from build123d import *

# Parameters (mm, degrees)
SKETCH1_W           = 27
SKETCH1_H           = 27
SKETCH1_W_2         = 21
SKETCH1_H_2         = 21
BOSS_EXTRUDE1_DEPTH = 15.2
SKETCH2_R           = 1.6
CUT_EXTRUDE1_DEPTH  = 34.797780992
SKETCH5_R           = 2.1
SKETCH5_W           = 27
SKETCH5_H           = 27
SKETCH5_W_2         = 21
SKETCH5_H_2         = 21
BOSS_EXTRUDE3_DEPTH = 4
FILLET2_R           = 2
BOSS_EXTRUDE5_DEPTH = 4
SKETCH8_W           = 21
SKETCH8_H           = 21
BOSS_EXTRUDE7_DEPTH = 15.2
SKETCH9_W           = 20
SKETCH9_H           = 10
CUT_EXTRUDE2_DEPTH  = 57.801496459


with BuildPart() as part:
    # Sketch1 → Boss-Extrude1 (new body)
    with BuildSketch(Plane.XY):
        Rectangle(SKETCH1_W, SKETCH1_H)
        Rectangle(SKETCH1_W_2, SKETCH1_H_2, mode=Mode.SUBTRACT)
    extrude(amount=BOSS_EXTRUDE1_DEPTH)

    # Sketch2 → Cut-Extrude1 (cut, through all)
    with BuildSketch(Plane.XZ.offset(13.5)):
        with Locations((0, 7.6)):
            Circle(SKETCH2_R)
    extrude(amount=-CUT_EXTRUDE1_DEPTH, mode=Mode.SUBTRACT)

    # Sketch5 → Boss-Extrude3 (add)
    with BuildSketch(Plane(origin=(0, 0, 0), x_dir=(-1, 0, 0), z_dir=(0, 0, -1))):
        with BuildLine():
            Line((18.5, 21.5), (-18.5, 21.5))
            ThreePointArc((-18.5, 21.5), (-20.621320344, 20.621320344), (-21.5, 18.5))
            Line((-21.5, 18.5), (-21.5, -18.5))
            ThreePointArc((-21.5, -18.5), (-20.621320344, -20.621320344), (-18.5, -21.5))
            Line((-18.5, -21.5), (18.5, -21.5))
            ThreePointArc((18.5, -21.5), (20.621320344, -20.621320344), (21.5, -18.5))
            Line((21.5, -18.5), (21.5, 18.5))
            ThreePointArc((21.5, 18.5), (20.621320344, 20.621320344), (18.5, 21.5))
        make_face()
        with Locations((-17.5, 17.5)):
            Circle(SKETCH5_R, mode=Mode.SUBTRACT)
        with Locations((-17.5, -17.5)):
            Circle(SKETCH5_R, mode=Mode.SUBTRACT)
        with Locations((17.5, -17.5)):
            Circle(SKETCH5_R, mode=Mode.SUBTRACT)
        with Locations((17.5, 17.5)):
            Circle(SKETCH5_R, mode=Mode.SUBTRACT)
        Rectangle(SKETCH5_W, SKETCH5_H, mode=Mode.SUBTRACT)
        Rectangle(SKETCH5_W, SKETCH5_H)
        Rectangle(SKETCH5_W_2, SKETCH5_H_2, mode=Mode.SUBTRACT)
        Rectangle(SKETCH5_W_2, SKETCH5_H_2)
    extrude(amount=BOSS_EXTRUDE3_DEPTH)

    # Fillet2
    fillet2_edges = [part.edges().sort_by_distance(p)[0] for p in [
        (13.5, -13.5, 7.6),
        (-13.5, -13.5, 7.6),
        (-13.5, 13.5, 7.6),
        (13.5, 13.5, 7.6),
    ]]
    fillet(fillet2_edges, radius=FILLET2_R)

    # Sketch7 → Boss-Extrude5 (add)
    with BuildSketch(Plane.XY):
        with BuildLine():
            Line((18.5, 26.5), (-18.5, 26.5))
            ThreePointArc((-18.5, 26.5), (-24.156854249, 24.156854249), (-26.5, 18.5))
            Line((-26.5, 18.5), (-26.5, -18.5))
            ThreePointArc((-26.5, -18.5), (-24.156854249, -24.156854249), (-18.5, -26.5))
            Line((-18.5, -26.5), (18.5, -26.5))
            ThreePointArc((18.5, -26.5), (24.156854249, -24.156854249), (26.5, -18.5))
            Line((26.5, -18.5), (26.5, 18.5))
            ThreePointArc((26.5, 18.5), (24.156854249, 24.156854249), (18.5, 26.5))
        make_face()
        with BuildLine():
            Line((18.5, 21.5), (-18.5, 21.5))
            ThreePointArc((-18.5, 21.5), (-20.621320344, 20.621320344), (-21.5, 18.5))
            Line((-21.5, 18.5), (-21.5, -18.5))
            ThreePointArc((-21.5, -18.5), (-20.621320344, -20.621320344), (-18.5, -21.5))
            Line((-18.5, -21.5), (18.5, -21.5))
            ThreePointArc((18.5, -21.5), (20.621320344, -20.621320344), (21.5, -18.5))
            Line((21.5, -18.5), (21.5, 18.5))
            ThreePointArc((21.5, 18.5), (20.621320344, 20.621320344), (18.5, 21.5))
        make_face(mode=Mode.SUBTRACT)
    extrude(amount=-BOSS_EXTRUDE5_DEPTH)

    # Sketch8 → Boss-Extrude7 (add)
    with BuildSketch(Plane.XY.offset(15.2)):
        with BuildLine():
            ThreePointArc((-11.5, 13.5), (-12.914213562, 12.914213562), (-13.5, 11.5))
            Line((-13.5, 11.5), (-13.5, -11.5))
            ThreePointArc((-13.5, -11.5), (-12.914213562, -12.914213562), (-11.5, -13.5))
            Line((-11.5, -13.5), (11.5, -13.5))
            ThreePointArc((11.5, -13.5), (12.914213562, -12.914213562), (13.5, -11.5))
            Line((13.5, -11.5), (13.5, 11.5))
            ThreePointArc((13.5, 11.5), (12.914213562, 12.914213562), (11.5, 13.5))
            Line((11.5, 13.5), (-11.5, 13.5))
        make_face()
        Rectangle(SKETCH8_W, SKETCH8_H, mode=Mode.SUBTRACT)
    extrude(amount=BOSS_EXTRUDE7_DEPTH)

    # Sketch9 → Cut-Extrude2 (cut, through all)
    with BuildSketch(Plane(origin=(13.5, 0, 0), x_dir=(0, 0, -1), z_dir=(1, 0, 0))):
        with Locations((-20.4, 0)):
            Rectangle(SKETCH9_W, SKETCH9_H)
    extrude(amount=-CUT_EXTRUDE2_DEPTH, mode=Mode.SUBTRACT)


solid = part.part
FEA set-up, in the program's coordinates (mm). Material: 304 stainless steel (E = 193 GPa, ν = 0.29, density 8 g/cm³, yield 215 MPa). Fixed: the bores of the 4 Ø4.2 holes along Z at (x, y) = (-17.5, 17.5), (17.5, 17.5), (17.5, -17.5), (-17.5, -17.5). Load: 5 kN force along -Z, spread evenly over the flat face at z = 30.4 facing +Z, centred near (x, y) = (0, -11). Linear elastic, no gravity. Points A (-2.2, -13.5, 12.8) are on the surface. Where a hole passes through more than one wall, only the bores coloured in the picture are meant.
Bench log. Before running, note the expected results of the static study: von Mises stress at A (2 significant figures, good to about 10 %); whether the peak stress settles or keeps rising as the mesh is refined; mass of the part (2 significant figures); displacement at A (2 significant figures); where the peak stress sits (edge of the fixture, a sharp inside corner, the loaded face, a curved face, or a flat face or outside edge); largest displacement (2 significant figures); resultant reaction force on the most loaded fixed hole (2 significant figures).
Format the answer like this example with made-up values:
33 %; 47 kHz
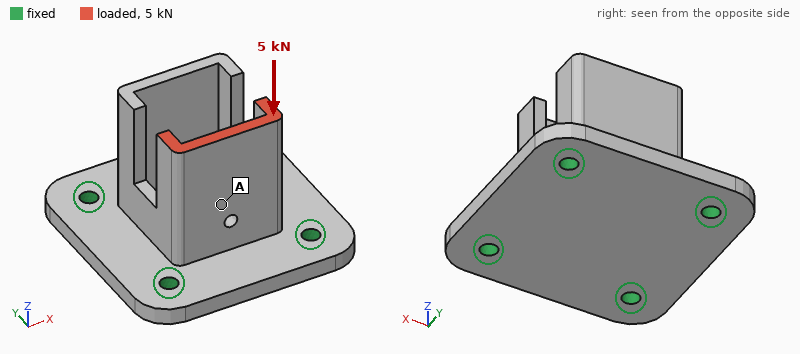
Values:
36 MPa; keeps rising; 150 g; 19 µm; edge of the fixture; 29 µm; 2.2 kN
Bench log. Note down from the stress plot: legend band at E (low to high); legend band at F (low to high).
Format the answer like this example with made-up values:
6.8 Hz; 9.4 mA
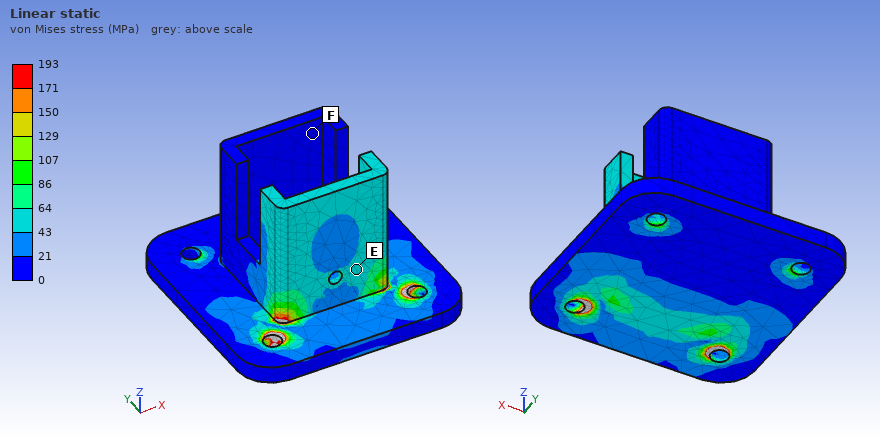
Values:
43 to 64 MPa; 0 to 21 MPa
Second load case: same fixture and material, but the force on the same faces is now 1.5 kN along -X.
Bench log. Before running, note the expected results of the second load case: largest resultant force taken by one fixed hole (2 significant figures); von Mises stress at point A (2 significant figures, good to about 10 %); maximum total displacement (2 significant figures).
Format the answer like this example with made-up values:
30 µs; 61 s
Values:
1.5 kN; 22 MPa; 65 µm
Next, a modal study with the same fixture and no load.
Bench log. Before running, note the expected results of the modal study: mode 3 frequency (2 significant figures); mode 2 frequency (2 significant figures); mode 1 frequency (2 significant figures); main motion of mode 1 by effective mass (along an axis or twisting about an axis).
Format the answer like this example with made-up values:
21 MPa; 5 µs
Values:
8400 Hz; 7300 Hz; 6600 Hz; along Y
